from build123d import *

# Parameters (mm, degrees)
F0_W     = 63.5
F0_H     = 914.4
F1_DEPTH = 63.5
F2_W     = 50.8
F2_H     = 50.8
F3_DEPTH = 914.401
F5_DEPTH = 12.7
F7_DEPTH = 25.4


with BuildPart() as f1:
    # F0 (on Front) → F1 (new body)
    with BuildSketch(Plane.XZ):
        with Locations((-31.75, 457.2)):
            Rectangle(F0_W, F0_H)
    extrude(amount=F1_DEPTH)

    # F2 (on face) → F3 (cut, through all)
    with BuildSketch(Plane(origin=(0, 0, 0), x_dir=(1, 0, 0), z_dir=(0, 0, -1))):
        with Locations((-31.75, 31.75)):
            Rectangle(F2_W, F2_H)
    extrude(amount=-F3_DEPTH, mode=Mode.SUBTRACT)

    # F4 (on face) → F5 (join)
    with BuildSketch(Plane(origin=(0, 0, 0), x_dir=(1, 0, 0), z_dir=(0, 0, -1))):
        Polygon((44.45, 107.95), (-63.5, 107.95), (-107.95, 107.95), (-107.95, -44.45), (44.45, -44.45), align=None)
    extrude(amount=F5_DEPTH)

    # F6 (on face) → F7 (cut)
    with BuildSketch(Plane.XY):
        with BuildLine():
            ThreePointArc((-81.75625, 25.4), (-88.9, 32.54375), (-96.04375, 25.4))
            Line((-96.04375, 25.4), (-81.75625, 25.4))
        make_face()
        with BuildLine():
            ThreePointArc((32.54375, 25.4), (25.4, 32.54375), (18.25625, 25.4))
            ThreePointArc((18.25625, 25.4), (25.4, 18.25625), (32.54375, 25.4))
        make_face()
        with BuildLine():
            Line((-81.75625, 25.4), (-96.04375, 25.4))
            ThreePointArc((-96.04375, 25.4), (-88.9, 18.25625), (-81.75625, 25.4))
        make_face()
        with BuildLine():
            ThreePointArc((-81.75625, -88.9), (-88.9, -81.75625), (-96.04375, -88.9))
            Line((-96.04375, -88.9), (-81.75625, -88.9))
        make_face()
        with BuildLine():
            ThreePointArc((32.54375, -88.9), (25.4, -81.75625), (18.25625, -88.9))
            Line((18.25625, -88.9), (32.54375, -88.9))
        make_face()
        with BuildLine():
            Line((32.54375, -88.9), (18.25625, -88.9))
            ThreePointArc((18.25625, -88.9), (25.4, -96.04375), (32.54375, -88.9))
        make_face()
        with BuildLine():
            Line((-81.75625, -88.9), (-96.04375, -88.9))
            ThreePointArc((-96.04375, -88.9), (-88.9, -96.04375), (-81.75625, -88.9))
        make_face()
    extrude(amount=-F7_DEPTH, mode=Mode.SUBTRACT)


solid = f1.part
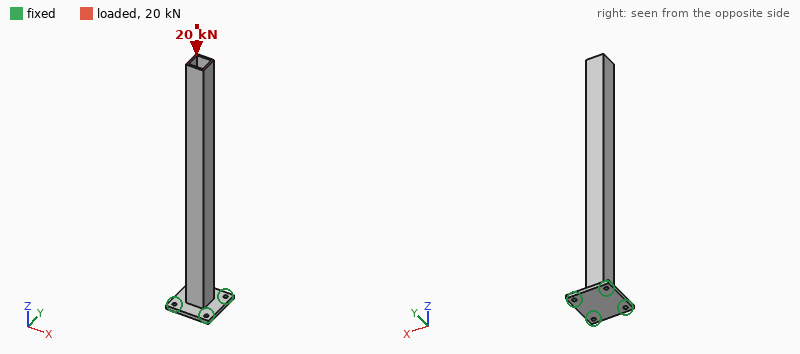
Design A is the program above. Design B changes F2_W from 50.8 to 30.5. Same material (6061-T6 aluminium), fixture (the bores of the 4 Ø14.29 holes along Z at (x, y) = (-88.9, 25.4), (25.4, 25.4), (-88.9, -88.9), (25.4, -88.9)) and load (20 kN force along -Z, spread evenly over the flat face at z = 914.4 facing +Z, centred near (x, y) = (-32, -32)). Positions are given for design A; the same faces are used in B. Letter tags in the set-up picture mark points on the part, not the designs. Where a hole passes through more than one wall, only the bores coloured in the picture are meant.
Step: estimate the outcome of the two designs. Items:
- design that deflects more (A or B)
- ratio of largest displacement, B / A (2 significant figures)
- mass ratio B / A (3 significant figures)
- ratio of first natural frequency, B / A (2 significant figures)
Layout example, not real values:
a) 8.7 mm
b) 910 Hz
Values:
a) A
b) 0.69
c) 1.58
d) 0.84
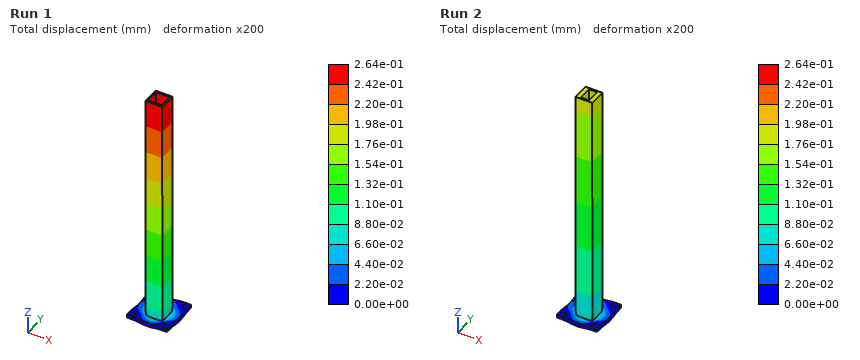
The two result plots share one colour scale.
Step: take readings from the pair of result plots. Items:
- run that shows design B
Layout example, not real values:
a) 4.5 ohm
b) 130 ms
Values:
a) Run 2
